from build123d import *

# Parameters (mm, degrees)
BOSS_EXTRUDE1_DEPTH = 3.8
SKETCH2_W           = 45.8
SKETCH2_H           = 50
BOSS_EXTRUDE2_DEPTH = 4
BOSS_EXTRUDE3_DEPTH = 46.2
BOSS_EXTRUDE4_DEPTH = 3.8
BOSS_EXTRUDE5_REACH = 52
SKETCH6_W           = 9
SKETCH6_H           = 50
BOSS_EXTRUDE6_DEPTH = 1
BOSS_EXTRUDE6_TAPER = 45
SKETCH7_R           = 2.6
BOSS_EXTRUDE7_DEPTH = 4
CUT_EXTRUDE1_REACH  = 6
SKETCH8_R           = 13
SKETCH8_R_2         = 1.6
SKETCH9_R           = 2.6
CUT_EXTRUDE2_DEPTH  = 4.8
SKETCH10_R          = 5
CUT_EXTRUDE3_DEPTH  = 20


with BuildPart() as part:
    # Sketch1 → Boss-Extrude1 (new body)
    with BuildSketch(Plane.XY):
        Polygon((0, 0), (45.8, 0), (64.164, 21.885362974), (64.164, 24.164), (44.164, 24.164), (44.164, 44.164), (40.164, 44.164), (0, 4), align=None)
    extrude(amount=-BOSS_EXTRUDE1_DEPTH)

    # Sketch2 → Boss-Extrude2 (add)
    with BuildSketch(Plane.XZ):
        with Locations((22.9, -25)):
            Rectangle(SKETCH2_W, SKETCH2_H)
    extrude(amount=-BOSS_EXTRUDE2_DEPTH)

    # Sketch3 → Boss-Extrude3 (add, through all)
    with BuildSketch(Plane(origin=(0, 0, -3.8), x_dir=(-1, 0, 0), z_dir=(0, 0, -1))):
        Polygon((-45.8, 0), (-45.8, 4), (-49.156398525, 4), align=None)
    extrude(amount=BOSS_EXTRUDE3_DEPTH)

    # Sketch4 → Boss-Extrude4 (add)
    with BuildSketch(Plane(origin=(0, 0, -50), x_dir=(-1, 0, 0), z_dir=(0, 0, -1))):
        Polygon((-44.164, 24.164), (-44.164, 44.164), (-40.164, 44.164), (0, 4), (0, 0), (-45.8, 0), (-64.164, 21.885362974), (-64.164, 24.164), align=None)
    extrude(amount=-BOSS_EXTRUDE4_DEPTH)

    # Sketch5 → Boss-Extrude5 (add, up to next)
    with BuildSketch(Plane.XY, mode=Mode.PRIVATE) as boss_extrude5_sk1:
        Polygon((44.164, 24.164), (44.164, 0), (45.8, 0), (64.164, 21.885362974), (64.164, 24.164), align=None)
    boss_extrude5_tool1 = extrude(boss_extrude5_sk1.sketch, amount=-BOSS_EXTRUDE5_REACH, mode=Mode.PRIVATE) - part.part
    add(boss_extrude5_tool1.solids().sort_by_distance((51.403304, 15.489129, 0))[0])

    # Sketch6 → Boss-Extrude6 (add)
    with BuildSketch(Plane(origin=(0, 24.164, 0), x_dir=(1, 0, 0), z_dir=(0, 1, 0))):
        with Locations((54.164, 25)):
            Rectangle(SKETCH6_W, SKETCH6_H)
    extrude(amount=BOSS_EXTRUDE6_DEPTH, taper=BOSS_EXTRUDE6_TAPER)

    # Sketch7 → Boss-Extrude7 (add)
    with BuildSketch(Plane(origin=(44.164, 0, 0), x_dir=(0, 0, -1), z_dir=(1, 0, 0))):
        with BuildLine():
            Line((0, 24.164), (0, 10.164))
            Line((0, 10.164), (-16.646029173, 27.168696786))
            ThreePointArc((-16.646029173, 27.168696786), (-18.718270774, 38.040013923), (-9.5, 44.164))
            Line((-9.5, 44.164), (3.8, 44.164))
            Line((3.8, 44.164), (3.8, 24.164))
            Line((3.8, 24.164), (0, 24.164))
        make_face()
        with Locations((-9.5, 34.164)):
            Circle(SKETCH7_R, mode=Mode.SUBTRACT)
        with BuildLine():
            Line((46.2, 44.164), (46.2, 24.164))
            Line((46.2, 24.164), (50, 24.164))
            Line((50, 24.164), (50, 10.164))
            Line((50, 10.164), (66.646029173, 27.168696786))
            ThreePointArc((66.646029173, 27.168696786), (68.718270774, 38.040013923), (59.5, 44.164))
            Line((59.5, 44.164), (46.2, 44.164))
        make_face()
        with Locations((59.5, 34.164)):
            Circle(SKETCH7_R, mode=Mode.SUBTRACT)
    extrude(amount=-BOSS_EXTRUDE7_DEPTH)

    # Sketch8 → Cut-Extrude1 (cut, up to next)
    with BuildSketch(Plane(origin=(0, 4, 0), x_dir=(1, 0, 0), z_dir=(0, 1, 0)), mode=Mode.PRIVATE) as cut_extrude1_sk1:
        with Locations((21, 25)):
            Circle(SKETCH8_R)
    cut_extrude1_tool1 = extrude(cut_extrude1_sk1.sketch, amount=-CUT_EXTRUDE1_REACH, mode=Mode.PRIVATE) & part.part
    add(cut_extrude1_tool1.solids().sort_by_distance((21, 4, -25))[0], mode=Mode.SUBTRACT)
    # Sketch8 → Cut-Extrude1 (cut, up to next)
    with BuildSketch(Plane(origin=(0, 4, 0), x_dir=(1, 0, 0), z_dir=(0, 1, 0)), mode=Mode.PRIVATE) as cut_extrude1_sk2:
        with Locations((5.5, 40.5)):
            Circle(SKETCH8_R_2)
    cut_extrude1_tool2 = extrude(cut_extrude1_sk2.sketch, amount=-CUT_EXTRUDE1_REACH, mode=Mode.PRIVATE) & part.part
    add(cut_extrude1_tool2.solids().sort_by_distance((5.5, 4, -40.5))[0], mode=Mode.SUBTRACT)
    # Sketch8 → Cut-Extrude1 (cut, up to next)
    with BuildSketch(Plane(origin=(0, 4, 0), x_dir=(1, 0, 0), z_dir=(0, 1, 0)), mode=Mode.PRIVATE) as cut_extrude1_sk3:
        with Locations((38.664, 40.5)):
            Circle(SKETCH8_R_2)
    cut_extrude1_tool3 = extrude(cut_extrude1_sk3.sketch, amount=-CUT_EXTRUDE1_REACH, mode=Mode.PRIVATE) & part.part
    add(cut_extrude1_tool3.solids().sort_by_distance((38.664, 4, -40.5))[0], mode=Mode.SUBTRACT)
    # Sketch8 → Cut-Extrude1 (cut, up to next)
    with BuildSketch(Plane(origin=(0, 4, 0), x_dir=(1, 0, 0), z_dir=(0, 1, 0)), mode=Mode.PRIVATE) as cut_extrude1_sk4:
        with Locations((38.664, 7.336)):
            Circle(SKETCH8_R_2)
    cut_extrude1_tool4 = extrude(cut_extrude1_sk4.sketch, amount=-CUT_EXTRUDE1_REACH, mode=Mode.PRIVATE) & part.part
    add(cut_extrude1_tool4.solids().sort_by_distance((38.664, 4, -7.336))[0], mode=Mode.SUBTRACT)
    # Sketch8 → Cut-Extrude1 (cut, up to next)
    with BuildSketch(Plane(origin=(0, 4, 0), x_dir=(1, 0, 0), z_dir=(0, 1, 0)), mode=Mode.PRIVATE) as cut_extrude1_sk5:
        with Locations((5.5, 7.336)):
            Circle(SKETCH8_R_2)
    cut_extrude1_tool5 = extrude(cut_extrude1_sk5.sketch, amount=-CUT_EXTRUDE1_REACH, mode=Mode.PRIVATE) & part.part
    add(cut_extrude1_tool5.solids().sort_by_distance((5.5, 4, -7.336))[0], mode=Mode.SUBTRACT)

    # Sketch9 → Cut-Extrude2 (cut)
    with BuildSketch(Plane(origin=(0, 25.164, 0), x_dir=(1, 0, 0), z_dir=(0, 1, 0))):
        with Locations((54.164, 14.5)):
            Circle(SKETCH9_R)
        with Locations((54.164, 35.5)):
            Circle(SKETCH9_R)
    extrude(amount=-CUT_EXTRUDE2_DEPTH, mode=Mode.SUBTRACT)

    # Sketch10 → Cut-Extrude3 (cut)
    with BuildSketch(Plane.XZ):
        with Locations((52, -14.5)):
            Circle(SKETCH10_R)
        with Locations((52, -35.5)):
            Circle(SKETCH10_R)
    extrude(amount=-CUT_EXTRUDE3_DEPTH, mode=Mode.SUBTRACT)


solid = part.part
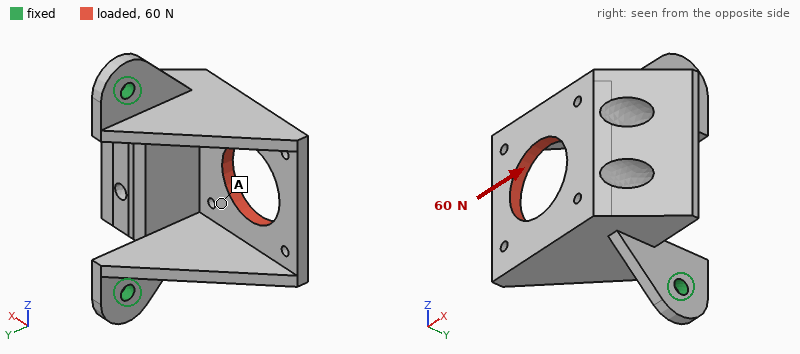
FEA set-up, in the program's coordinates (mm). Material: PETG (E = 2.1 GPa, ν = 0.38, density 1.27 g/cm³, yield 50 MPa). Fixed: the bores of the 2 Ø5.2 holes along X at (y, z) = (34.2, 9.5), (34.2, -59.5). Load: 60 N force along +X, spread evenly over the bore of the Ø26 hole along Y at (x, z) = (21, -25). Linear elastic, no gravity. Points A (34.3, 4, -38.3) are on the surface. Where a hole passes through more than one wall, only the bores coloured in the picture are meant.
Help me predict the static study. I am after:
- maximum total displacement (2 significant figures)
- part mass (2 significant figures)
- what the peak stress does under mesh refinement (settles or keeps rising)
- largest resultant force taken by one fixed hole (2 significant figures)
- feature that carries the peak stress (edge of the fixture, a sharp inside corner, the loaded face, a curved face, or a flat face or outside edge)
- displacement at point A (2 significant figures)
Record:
1.1 mm
38 g
keeps rising
31 N
edge of the fixture
0.63 mm
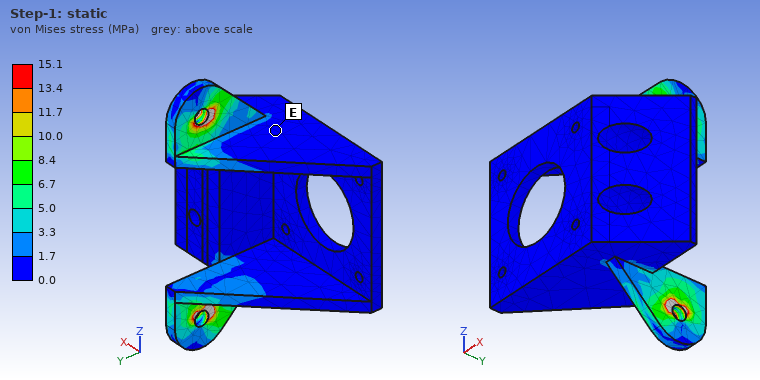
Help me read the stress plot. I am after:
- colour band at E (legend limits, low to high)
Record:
0.0 to 1.7 MPa
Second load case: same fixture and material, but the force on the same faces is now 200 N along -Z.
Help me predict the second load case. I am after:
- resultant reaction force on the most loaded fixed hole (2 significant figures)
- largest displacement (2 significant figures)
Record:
140 N
1.00 mm
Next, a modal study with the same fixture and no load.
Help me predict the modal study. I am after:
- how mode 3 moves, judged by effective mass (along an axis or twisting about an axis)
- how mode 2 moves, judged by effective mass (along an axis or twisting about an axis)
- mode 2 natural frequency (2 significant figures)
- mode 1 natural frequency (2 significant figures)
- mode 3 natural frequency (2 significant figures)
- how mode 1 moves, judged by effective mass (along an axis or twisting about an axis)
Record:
along X
along Z
680 Hz
300 Hz
1400 Hz
along X
